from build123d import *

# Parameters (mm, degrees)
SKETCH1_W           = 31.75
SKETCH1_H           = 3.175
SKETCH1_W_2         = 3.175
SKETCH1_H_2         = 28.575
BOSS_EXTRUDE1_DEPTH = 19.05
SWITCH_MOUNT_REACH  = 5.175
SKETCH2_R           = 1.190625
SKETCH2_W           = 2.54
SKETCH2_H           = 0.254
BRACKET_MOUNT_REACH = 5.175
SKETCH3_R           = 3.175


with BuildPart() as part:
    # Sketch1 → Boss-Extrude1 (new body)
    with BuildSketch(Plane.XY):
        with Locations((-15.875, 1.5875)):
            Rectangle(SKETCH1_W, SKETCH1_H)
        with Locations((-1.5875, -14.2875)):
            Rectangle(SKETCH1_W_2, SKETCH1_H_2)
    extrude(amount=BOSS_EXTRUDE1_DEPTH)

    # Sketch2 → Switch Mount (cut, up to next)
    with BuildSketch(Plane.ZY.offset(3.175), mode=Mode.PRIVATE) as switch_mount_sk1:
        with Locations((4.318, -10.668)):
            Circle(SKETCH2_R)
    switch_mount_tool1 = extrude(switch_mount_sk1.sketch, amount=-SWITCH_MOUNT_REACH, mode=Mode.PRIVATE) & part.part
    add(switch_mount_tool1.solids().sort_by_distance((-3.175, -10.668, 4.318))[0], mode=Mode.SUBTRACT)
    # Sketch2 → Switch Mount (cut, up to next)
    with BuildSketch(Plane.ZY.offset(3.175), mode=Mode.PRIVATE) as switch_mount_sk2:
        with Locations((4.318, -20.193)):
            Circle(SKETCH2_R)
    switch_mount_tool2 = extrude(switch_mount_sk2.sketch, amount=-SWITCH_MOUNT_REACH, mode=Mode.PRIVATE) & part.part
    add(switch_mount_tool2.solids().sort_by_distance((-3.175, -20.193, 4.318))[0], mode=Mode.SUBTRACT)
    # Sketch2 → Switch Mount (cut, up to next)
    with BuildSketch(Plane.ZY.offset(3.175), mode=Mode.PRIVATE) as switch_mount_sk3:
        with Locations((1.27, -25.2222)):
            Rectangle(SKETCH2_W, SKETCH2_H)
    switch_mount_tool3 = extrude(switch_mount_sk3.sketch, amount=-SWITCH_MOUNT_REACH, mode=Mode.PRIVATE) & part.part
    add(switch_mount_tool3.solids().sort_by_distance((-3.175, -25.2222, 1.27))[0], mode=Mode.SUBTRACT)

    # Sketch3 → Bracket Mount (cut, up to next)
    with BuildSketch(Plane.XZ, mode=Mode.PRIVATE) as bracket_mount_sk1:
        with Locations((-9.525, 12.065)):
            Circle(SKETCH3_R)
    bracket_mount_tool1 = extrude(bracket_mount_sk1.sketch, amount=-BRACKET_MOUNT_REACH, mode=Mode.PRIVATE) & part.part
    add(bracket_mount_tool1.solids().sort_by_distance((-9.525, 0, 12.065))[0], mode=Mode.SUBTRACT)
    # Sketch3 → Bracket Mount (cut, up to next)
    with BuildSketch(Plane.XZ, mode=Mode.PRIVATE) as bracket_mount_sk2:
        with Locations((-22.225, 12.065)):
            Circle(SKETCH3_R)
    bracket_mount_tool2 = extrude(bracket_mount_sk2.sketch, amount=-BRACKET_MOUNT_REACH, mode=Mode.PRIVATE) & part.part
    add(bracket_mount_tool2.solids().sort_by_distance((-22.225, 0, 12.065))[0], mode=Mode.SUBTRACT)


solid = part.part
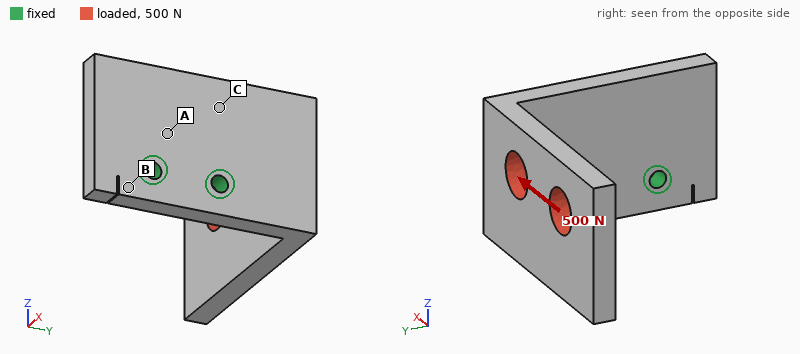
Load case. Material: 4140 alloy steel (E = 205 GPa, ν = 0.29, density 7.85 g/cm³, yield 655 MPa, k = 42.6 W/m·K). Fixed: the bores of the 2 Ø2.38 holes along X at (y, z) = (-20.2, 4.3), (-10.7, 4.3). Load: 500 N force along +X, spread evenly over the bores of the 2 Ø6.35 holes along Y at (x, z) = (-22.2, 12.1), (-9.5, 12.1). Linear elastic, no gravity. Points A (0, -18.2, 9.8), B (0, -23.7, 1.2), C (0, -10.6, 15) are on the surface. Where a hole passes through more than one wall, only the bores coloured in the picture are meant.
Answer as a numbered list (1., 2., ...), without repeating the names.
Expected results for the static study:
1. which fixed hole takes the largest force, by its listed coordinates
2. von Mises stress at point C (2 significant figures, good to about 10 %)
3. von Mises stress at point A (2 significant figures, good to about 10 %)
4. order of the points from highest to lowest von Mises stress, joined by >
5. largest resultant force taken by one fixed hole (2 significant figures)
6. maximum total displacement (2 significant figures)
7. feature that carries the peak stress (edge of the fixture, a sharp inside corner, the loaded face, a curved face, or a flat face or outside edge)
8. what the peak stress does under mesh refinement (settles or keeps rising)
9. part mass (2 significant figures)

1. (-10.7, 4.3)
2. 110 MPa
3. 56 MPa
4. C > A > B
5. 750 N
6. 0.19 mm
7. edge of the fixture
8. keeps rising
9. 27 g
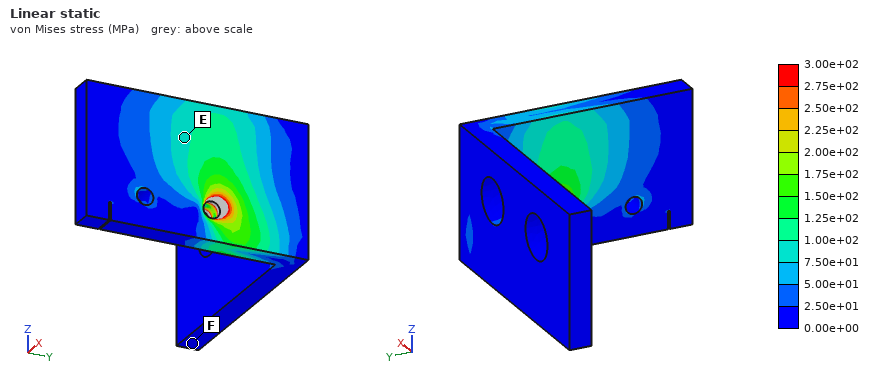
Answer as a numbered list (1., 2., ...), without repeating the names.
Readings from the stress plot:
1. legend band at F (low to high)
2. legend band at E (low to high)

1. 0.00e+00 to 2.50e+01 MPa
2. 7.50e+01 to 1.00e+02 MPa
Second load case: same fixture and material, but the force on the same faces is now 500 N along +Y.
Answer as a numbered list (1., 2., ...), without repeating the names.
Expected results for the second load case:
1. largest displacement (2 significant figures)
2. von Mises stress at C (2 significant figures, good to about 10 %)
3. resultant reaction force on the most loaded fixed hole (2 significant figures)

1. 0.45 mm
2. 130 MPa
3. 550 N
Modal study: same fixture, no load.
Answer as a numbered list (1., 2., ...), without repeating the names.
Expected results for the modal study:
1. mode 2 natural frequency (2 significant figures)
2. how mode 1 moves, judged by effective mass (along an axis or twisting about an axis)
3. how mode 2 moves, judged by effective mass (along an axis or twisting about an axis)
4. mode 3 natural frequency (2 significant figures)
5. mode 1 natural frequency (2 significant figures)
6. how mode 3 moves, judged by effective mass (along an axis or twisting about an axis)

1. 2500 Hz
2. along Y
3. along Z
4. 6200 Hz
5. 1700 Hz
6. along X
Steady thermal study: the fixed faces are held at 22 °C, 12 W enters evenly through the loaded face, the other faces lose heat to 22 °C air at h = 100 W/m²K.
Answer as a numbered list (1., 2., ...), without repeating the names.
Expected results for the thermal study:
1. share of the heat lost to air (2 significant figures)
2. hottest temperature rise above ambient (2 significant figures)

1. 63 %
2. 66 K
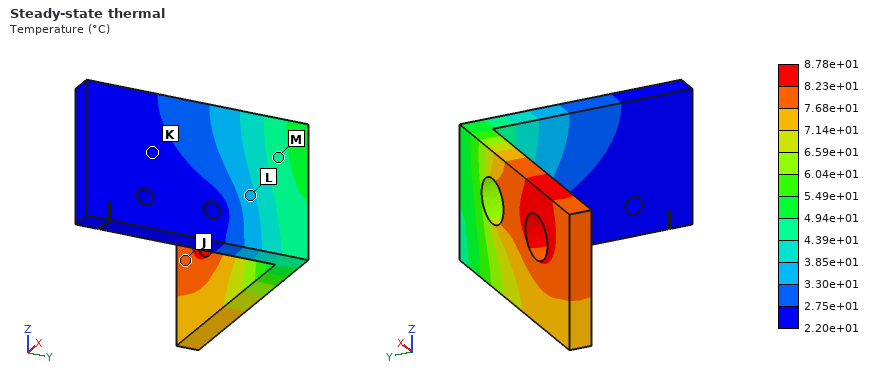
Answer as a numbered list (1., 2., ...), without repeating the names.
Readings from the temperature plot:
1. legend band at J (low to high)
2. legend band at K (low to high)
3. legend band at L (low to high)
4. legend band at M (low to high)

1. 7.68e+01 to 8.23e+01 °C
2. 2.20e+01 to 2.75e+01 °C
3. 3.30e+01 to 3.85e+01 °C
4. 4.39e+01 to 4.94e+01 °C
